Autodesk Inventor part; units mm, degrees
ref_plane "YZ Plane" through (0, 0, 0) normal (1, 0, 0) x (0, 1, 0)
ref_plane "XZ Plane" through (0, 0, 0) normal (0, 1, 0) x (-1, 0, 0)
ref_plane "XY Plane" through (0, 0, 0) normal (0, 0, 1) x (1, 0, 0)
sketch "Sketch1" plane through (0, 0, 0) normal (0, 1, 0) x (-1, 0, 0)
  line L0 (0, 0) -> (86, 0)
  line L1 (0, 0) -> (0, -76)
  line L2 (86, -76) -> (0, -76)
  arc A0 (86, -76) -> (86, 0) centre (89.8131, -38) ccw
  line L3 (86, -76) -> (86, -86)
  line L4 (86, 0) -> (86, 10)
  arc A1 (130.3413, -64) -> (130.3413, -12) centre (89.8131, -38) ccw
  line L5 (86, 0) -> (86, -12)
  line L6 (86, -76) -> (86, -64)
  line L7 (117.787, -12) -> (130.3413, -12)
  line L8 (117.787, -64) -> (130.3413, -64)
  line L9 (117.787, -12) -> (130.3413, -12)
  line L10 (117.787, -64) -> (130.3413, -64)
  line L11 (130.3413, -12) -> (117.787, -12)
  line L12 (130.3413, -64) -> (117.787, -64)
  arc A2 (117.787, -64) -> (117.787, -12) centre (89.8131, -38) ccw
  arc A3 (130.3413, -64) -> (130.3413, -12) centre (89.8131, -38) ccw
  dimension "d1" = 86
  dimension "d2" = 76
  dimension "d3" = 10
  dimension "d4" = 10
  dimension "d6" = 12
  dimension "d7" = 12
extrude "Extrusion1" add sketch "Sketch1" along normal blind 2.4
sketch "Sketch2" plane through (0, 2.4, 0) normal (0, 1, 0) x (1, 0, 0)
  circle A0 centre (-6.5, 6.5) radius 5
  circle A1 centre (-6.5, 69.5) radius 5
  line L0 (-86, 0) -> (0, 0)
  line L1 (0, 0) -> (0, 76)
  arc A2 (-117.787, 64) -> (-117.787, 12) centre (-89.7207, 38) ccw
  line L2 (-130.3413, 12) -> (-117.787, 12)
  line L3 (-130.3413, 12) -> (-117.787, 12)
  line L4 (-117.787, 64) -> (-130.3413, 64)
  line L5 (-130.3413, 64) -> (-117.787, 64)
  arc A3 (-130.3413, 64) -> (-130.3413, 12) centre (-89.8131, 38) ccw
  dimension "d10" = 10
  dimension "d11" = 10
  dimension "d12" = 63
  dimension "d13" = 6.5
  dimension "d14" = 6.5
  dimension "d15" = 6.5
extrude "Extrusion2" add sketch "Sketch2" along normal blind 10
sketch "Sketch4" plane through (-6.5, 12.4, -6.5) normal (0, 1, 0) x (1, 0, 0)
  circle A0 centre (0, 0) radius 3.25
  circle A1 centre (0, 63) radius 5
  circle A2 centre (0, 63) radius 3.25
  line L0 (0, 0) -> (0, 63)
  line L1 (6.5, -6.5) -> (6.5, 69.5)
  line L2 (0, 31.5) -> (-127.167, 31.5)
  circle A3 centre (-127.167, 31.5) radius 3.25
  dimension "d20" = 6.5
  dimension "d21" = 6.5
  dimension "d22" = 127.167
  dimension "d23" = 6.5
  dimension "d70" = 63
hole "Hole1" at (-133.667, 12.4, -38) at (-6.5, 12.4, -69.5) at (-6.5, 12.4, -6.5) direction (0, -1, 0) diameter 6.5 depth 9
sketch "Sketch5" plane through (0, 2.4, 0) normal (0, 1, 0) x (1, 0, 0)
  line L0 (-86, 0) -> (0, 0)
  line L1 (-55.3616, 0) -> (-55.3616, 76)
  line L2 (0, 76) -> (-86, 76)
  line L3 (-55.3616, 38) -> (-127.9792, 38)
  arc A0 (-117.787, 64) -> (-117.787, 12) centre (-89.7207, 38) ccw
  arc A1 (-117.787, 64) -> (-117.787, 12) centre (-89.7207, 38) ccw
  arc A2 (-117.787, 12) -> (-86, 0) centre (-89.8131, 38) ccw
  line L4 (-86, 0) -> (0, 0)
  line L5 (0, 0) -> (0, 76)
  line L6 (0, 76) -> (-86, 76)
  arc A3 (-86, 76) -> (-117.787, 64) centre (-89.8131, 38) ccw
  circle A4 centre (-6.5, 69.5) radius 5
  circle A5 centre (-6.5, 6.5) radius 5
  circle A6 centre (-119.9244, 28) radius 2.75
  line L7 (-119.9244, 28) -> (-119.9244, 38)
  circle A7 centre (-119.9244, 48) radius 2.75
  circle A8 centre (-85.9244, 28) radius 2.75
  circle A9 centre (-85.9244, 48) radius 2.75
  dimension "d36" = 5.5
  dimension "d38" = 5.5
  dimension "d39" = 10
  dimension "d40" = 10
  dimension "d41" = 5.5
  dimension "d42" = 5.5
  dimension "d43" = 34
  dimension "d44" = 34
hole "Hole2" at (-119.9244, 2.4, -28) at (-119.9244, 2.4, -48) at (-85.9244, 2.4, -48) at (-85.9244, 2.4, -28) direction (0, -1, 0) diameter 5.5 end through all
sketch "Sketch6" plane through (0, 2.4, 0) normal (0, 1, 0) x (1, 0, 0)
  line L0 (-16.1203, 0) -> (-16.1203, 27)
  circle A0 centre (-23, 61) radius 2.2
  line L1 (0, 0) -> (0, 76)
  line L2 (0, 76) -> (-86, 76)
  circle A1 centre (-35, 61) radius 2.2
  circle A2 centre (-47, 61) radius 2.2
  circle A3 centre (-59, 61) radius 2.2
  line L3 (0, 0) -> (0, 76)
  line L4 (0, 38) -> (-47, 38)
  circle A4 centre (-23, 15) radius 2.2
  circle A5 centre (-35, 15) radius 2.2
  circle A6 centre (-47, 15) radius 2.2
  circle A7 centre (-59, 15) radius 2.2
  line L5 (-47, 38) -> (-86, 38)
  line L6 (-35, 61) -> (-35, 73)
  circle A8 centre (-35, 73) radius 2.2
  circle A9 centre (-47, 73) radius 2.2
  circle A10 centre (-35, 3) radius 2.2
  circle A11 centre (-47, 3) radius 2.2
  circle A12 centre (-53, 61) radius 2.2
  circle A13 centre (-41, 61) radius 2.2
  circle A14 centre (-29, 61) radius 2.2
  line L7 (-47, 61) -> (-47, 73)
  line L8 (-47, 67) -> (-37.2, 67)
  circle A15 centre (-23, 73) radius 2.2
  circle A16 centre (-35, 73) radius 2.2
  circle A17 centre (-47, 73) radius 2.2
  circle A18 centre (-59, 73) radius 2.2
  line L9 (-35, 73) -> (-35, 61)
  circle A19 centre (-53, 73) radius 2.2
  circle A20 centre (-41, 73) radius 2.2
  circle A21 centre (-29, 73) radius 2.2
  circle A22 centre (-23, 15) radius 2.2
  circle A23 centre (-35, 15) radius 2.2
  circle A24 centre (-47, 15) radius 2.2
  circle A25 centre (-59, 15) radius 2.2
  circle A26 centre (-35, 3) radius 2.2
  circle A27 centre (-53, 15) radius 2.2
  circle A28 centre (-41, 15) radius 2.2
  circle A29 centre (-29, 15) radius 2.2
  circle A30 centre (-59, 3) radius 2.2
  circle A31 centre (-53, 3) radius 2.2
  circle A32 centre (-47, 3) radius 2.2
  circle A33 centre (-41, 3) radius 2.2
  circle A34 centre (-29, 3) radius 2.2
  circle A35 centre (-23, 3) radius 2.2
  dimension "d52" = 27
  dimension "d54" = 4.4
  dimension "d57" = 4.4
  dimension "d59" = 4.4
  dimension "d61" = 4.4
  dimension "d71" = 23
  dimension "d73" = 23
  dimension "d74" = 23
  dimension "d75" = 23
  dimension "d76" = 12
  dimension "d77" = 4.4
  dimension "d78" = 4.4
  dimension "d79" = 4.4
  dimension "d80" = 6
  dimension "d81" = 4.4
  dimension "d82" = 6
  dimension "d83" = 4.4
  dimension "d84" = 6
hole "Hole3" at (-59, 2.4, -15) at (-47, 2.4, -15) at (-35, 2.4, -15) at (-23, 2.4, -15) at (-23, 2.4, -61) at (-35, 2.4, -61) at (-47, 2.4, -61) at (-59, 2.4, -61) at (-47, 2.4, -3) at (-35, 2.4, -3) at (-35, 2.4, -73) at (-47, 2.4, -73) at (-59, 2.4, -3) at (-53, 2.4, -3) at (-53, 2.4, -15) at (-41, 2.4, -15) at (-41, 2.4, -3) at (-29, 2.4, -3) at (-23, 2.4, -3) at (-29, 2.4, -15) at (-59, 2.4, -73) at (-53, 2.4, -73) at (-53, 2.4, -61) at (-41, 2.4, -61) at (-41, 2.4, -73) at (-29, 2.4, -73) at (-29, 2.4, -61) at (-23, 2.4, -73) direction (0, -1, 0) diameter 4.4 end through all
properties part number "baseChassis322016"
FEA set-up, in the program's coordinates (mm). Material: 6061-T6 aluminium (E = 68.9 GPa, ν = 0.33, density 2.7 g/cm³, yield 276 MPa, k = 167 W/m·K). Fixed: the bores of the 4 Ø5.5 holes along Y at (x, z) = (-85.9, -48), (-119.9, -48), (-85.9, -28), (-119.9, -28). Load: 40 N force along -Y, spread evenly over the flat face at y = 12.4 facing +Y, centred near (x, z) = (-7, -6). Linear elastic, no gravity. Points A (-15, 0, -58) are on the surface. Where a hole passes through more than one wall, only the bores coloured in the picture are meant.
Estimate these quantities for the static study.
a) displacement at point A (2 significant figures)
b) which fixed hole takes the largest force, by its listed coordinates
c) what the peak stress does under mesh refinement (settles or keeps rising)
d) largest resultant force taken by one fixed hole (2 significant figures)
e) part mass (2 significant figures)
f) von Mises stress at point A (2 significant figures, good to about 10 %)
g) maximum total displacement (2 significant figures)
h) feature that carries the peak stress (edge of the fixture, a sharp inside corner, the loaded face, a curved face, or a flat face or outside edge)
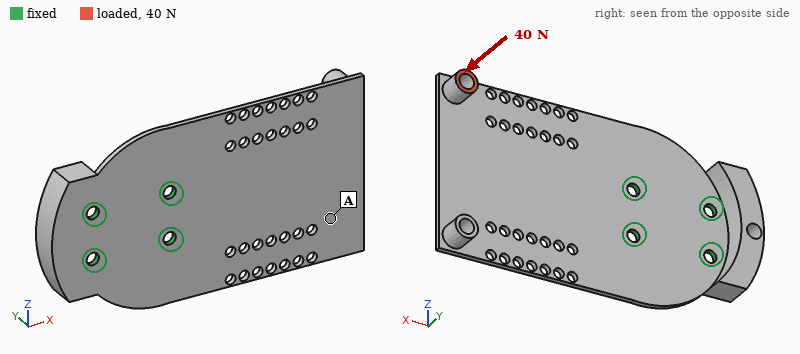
0.79 mm
(-85.9, -28)
keeps rising
76 N
76 g
9.0 MPa
1.7 mm
edge of the fixture
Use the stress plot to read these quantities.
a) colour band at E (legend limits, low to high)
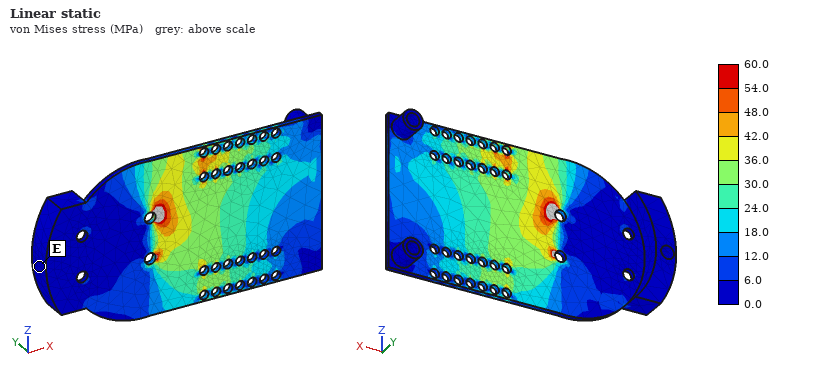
0.0 to 6.0 MPa
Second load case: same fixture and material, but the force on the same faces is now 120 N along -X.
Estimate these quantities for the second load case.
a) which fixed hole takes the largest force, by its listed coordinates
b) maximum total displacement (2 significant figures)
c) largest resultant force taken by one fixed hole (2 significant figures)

(-85.9, -28)
1.1 mm
120 N
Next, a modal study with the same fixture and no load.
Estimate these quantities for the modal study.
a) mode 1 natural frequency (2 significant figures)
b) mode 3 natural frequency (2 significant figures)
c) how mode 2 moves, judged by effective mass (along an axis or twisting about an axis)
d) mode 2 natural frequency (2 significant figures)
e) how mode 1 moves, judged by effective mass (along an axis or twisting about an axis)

240 Hz
1500 Hz
twisting about X
560 Hz
along Y
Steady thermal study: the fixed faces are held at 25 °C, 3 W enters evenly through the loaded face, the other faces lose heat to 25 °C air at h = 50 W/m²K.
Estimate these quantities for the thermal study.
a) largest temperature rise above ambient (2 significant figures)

13 K
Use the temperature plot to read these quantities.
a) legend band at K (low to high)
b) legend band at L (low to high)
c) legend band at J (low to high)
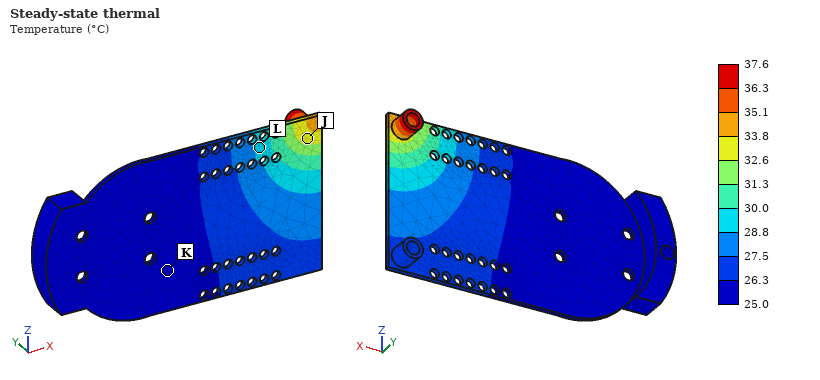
25.0 to 26.3 °C
28.8 to 30.0 °C
32.6 to 33.8 °C
